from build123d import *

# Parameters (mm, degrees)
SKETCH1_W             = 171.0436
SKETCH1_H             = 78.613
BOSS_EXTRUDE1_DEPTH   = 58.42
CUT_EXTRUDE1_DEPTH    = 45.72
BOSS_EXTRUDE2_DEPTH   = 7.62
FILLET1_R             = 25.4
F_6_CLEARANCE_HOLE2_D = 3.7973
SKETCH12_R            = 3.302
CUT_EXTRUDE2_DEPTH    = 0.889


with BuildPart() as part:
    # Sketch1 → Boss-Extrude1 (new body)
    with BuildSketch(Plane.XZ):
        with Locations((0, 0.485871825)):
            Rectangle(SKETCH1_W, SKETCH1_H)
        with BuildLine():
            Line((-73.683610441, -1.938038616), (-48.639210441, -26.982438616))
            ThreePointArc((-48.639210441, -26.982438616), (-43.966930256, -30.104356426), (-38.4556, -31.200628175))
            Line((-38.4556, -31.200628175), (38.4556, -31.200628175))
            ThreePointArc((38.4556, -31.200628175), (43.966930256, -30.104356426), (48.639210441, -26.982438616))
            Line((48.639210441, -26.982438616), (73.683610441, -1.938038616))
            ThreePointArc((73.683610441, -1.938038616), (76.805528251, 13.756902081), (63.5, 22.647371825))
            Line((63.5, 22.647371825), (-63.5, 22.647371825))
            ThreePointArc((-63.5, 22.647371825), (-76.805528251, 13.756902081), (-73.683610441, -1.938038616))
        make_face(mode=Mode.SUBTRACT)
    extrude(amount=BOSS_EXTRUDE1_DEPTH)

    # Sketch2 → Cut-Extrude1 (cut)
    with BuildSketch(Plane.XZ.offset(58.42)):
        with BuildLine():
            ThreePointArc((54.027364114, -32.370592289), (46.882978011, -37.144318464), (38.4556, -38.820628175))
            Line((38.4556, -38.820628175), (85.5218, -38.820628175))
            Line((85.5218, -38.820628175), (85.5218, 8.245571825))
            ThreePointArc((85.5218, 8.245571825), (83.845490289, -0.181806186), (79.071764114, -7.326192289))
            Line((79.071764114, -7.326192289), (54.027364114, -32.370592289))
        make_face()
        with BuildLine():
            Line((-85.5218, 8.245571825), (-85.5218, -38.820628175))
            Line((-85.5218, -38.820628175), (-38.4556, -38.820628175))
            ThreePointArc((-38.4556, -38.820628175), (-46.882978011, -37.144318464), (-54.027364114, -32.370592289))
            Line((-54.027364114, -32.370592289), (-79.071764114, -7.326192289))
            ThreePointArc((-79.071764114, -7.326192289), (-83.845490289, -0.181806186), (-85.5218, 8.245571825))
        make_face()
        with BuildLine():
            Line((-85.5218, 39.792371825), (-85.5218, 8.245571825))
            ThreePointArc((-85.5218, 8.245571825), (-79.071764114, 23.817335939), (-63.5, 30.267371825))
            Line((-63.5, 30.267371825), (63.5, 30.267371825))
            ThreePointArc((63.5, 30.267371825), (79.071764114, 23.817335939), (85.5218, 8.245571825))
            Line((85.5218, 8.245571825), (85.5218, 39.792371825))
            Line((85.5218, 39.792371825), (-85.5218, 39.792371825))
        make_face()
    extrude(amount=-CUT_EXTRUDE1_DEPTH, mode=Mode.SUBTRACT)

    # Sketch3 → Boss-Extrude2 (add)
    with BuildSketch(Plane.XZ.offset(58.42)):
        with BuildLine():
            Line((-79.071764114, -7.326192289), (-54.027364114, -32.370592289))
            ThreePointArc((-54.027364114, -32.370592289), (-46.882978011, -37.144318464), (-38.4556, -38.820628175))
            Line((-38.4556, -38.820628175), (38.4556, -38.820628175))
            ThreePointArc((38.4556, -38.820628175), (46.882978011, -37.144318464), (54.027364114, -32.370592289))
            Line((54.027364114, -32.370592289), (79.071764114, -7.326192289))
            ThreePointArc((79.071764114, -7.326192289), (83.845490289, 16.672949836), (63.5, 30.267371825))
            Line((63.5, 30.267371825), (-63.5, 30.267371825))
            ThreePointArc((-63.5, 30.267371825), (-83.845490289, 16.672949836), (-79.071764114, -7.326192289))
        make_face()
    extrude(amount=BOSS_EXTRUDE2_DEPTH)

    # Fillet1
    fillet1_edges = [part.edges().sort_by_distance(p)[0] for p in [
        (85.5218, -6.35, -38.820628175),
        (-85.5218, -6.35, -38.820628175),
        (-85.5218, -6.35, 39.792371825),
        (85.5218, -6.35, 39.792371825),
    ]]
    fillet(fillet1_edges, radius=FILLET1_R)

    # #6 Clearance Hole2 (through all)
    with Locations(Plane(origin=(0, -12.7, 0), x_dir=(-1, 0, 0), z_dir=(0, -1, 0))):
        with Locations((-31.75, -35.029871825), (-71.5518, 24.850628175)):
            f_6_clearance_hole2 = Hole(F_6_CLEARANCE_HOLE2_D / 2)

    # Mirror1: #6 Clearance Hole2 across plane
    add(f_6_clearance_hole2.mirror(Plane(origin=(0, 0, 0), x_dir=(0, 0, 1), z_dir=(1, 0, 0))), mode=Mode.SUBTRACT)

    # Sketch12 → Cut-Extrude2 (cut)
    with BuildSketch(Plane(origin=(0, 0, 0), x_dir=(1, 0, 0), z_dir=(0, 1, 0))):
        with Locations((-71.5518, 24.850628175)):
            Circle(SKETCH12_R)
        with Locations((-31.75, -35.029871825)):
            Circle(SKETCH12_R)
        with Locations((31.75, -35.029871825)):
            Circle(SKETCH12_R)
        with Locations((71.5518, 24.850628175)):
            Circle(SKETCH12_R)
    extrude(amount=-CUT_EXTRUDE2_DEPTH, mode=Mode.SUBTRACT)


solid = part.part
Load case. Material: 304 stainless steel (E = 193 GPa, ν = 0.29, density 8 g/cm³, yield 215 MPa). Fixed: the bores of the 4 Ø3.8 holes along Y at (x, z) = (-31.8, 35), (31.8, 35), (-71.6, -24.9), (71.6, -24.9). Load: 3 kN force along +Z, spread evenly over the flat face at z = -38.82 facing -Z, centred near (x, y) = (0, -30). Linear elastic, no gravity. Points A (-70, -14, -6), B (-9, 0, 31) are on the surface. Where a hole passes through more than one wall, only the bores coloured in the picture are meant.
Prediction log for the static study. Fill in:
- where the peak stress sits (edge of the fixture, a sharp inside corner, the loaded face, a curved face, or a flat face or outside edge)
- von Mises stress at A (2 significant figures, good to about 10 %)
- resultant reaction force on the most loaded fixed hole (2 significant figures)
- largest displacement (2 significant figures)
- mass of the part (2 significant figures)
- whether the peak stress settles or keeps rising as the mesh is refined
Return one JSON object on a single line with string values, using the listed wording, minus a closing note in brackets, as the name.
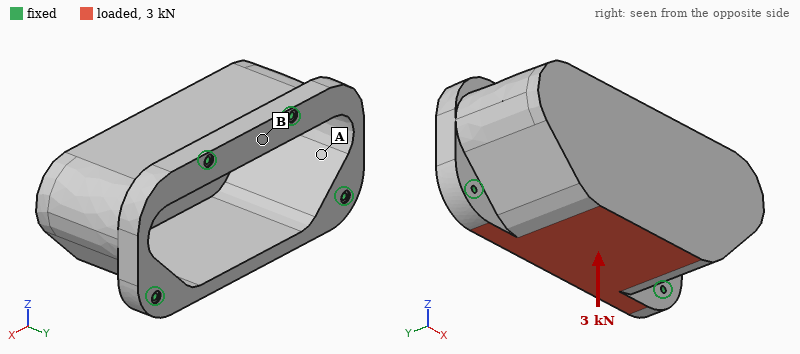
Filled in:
{"where the peak stress sits": "edge of the fixture", "von Mises stress at A": "6.4 MPa", "resultant reaction force on the most loaded fixed hole": "1.9 kN", "largest displacement": "26 µm", "mass of the part": "2.3 kg", "whether the peak stress settles or keeps rising as the mesh is refined": "keeps rising"}
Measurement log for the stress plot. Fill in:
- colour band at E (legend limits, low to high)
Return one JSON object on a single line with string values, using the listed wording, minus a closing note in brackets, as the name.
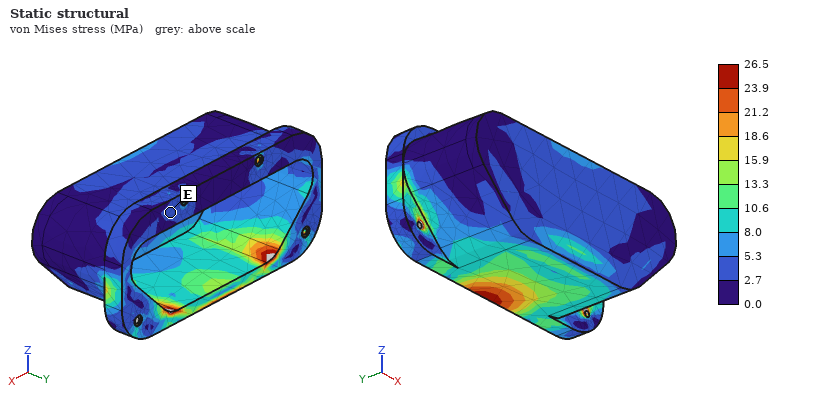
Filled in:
{"colour band at E": "2.7 to 5.3 MPa"}
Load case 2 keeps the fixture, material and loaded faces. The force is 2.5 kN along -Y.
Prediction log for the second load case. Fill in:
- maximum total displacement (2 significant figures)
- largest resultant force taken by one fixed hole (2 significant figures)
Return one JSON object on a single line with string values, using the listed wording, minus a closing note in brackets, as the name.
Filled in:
{"maximum total displacement": "7.2 µm", "largest resultant force taken by one fixed hole": "1.7 kN"}
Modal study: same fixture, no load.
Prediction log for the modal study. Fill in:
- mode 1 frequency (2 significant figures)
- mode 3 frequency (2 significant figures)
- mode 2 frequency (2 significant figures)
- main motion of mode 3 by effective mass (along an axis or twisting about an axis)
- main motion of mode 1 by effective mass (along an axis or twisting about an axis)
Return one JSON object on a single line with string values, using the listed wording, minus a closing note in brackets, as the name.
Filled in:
{"mode 1 frequency": "2400 Hz", "mode 3 frequency": "4200 Hz", "mode 2 frequency": "4000 Hz", "main motion of mode 3 by effective mass": "along X", "main motion of mode 1 by effective mass": "along Z"}
